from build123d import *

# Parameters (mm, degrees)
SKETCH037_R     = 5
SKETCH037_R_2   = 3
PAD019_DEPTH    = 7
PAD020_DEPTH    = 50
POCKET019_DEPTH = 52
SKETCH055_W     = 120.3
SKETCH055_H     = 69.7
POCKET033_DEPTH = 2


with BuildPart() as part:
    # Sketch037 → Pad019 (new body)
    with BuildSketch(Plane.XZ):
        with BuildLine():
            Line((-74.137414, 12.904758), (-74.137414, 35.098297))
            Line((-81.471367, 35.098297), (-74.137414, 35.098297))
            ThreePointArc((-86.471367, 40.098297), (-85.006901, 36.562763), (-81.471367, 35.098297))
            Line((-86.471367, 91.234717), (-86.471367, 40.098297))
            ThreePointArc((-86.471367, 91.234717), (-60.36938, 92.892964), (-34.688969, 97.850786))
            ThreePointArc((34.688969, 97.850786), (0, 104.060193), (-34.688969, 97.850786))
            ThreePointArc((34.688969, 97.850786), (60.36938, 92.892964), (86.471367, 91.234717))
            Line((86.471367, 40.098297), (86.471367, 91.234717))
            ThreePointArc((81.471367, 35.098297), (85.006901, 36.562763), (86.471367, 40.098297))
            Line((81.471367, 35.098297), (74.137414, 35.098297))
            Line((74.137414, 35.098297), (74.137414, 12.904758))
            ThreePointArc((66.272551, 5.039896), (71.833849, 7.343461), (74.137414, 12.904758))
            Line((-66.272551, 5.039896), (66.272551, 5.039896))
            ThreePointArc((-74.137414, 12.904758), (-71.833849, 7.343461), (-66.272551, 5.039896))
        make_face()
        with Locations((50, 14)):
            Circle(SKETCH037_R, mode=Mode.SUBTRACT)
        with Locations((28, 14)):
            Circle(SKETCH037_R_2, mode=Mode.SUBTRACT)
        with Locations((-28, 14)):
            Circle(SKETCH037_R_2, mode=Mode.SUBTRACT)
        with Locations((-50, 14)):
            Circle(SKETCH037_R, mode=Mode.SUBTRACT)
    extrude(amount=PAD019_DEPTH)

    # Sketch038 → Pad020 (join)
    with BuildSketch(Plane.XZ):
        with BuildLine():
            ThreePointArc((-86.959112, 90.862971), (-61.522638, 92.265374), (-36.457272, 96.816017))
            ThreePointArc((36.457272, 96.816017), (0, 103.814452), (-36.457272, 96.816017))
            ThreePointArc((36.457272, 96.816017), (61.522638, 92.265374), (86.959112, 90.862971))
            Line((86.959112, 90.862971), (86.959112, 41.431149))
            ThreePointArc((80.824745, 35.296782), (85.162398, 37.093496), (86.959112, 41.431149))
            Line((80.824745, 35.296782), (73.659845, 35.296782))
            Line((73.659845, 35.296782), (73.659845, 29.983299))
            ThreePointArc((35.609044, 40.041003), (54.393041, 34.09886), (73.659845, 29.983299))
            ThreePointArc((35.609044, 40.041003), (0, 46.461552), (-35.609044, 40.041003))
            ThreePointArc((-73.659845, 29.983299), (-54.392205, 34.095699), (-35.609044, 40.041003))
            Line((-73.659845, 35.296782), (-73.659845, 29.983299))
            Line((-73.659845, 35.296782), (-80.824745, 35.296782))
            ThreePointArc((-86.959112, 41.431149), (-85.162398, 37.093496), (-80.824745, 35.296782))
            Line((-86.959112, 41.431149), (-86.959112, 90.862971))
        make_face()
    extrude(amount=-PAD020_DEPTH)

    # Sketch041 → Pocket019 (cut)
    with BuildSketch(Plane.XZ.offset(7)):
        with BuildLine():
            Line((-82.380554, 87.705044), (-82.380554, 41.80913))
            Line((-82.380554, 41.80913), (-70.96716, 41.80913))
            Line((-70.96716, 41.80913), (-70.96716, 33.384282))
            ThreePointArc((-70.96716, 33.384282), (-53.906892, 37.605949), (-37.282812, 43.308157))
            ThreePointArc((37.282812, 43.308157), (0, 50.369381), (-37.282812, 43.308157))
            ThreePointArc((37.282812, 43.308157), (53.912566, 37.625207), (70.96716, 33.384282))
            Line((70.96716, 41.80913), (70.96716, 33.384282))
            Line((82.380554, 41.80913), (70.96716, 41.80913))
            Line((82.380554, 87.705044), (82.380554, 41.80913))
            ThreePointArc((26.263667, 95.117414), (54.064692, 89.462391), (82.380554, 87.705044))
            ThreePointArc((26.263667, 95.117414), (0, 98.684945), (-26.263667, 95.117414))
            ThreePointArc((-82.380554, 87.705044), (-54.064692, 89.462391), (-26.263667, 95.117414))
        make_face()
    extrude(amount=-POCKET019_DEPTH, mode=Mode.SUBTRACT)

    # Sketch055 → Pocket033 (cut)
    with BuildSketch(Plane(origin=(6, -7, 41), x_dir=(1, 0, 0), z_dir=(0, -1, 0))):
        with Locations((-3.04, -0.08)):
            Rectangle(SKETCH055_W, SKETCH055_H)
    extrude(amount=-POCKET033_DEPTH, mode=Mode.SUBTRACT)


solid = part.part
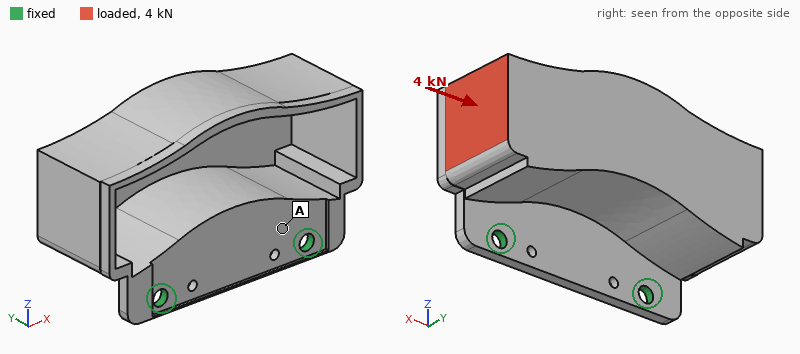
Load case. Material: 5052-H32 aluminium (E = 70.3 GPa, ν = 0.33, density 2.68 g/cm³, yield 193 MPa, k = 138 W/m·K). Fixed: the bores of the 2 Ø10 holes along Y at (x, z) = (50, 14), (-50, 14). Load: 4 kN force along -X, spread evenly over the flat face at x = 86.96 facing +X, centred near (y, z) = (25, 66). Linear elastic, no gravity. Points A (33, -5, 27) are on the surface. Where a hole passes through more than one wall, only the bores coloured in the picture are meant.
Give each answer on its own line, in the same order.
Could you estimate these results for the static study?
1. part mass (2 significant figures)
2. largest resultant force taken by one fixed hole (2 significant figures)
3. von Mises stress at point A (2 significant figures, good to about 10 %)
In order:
470 g
3.0 kN
15 MPa
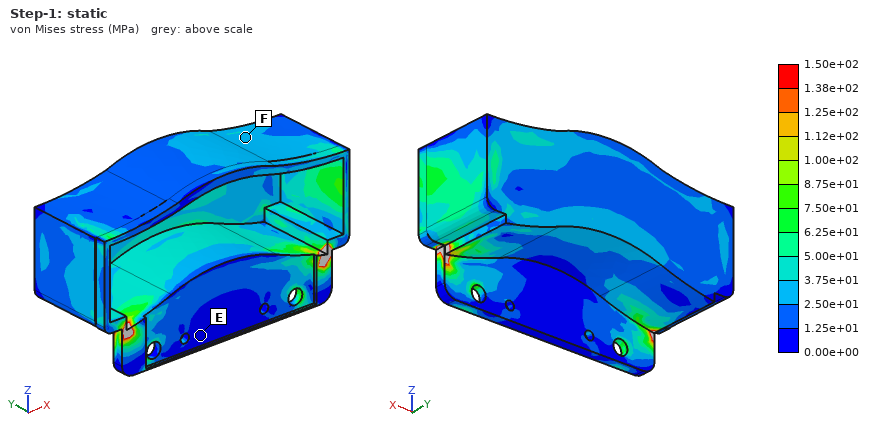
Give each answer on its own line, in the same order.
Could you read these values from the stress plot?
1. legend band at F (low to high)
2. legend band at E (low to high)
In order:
2.50e+01 to 3.75e+01 MPa
0.00e+00 to 1.25e+01 MPa
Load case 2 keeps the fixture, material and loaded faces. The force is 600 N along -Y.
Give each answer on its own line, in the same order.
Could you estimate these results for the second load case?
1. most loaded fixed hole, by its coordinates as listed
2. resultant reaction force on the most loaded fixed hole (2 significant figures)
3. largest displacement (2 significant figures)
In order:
(50, 14)
770 N
0.94 mm
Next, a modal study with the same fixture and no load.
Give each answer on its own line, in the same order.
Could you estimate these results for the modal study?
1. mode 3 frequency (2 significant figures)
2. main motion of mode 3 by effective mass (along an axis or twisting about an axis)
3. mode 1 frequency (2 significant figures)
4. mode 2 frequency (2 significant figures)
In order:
960 Hz
along Z
250 Hz
430 Hz
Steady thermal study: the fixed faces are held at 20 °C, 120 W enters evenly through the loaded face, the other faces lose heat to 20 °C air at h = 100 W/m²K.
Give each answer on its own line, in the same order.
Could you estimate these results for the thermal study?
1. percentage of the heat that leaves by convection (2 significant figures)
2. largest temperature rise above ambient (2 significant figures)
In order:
84 %
65 K
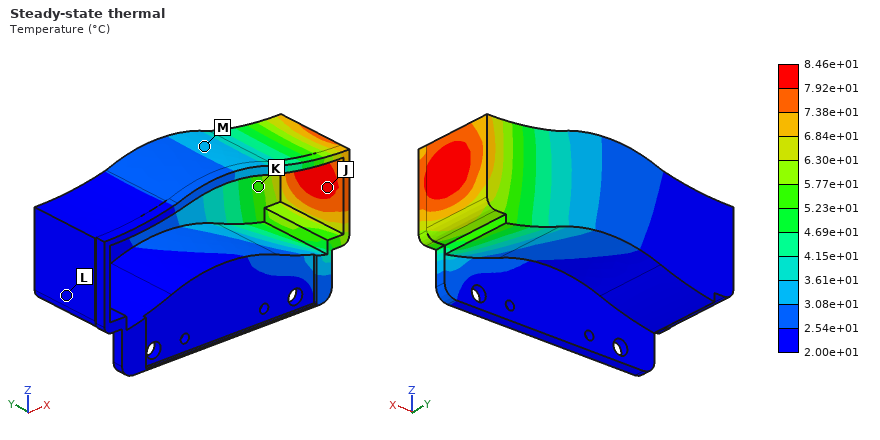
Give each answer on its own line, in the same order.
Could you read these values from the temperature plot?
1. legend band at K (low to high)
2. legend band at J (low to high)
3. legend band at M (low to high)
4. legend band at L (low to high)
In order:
5.23e+01 to 5.77e+01 °C
7.92e+01 to 8.46e+01 °C
3.08e+01 to 3.61e+01 °C
2.00e+01 to 2.54e+01 °C
